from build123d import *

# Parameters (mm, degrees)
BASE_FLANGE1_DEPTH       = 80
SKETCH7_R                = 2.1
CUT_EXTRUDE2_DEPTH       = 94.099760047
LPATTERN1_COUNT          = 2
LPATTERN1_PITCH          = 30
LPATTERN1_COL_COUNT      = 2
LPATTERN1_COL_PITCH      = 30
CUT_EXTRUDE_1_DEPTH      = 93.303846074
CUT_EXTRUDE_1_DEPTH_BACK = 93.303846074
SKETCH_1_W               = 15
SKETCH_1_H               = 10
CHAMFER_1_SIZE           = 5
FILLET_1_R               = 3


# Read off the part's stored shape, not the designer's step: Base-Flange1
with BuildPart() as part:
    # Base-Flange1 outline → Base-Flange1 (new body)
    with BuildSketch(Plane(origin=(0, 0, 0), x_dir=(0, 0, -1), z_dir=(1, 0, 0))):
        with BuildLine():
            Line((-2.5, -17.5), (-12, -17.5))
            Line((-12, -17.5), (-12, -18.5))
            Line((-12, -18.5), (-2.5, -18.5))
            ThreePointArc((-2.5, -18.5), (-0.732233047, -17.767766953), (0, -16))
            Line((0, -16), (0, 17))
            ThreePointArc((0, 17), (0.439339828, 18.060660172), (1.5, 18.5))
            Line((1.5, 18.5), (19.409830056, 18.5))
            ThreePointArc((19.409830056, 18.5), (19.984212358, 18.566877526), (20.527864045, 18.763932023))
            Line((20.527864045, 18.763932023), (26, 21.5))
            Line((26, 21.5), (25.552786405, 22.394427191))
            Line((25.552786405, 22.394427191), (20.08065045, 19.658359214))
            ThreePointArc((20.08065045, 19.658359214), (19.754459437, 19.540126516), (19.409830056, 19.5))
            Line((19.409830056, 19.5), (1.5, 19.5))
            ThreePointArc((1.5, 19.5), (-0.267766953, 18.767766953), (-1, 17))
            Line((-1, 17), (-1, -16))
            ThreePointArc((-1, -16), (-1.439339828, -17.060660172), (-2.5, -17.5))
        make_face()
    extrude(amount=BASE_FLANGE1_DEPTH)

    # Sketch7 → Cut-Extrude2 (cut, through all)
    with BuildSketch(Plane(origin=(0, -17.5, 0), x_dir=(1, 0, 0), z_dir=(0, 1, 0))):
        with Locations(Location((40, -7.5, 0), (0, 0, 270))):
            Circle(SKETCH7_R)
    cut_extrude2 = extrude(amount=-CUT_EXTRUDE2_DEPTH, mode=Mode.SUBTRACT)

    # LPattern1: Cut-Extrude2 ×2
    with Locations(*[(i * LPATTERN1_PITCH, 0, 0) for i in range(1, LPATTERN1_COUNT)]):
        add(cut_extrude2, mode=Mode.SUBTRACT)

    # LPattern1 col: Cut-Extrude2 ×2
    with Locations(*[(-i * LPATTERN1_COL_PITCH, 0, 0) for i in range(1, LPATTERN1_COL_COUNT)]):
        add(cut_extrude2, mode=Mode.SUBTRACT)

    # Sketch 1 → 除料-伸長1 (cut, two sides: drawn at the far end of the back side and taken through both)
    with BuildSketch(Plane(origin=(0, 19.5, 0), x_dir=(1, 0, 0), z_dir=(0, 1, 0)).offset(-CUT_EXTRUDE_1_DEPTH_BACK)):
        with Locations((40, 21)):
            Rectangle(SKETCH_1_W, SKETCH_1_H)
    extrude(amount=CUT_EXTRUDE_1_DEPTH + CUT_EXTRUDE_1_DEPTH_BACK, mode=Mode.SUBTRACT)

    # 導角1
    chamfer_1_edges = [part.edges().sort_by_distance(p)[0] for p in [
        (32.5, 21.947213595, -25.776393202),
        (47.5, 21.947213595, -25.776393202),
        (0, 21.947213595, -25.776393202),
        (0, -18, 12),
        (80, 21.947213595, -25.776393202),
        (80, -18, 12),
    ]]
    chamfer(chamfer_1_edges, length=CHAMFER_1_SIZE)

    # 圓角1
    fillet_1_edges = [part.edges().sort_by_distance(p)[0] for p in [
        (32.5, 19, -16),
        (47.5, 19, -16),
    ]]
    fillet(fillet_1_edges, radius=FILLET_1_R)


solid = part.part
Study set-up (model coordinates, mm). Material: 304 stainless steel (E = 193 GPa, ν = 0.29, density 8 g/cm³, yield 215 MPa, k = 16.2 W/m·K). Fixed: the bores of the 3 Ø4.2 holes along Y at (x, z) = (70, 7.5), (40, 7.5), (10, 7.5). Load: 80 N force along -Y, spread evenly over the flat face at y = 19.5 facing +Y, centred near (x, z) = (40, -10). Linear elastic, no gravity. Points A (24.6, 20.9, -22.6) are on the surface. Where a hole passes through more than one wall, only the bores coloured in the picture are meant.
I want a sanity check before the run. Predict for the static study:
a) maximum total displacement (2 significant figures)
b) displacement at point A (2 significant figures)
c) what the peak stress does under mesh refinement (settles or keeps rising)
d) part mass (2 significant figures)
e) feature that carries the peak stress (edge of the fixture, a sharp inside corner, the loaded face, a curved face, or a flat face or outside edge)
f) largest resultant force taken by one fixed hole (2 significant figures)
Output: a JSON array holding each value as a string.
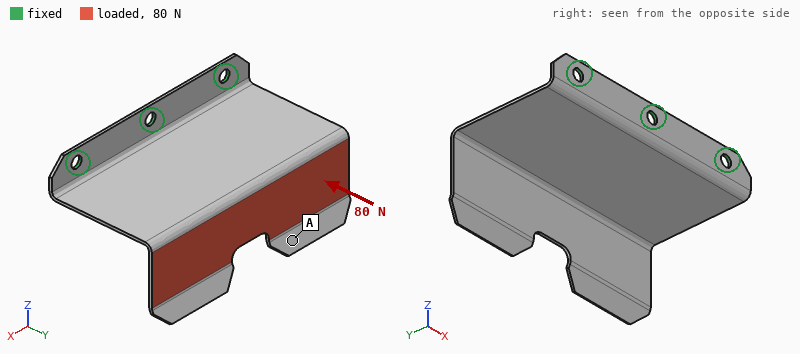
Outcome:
["1.1 mm", "1.0 mm", "keeps rising", "45 g", "edge of the fixture", "30 N"]
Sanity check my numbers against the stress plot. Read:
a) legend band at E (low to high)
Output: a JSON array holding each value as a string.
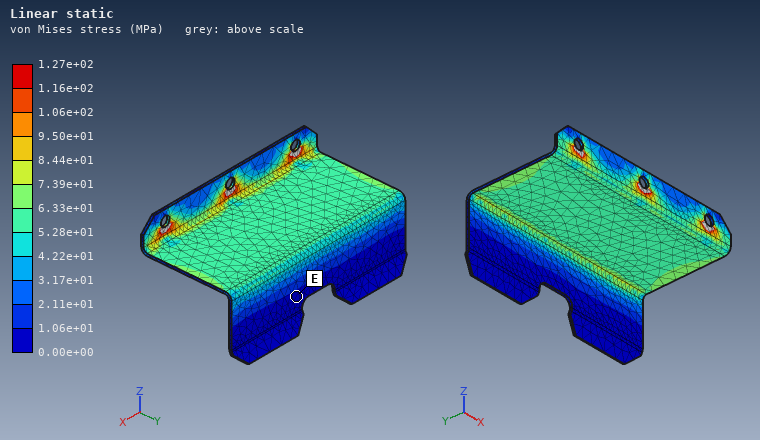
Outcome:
["0.00e+00 to 1.06e+01 MPa"]
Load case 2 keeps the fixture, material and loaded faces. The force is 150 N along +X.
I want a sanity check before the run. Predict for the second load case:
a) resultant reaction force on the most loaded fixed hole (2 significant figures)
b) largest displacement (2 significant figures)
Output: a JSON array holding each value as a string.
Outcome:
["110 N", "0.59 mm"]
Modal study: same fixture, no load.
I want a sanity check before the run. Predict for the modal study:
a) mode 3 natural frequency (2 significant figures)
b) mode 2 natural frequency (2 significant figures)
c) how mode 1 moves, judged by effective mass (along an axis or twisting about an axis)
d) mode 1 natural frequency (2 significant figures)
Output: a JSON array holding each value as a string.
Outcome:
["870 Hz", "420 Hz", "along Z", "230 Hz"]
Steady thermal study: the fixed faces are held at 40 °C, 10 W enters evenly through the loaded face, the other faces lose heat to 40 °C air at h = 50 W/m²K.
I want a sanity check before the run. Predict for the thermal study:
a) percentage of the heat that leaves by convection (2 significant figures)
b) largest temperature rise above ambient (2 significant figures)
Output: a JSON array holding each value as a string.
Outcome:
["98 %", "61 K"]
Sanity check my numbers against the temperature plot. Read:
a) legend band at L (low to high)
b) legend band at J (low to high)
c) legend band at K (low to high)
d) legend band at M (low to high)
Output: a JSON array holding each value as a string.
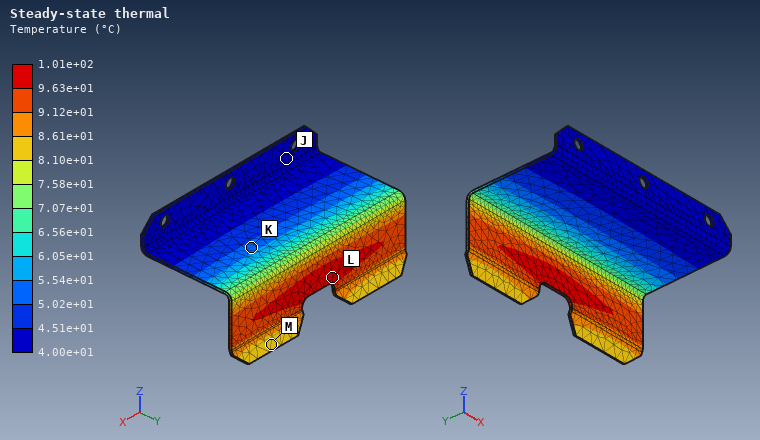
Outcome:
["9.63e+01 to 1.01e+02 °C", "4.00e+01 to 4.51e+01 °C", "5.02e+01 to 5.54e+01 °C", "8.10e+01 to 8.61e+01 °C"]
